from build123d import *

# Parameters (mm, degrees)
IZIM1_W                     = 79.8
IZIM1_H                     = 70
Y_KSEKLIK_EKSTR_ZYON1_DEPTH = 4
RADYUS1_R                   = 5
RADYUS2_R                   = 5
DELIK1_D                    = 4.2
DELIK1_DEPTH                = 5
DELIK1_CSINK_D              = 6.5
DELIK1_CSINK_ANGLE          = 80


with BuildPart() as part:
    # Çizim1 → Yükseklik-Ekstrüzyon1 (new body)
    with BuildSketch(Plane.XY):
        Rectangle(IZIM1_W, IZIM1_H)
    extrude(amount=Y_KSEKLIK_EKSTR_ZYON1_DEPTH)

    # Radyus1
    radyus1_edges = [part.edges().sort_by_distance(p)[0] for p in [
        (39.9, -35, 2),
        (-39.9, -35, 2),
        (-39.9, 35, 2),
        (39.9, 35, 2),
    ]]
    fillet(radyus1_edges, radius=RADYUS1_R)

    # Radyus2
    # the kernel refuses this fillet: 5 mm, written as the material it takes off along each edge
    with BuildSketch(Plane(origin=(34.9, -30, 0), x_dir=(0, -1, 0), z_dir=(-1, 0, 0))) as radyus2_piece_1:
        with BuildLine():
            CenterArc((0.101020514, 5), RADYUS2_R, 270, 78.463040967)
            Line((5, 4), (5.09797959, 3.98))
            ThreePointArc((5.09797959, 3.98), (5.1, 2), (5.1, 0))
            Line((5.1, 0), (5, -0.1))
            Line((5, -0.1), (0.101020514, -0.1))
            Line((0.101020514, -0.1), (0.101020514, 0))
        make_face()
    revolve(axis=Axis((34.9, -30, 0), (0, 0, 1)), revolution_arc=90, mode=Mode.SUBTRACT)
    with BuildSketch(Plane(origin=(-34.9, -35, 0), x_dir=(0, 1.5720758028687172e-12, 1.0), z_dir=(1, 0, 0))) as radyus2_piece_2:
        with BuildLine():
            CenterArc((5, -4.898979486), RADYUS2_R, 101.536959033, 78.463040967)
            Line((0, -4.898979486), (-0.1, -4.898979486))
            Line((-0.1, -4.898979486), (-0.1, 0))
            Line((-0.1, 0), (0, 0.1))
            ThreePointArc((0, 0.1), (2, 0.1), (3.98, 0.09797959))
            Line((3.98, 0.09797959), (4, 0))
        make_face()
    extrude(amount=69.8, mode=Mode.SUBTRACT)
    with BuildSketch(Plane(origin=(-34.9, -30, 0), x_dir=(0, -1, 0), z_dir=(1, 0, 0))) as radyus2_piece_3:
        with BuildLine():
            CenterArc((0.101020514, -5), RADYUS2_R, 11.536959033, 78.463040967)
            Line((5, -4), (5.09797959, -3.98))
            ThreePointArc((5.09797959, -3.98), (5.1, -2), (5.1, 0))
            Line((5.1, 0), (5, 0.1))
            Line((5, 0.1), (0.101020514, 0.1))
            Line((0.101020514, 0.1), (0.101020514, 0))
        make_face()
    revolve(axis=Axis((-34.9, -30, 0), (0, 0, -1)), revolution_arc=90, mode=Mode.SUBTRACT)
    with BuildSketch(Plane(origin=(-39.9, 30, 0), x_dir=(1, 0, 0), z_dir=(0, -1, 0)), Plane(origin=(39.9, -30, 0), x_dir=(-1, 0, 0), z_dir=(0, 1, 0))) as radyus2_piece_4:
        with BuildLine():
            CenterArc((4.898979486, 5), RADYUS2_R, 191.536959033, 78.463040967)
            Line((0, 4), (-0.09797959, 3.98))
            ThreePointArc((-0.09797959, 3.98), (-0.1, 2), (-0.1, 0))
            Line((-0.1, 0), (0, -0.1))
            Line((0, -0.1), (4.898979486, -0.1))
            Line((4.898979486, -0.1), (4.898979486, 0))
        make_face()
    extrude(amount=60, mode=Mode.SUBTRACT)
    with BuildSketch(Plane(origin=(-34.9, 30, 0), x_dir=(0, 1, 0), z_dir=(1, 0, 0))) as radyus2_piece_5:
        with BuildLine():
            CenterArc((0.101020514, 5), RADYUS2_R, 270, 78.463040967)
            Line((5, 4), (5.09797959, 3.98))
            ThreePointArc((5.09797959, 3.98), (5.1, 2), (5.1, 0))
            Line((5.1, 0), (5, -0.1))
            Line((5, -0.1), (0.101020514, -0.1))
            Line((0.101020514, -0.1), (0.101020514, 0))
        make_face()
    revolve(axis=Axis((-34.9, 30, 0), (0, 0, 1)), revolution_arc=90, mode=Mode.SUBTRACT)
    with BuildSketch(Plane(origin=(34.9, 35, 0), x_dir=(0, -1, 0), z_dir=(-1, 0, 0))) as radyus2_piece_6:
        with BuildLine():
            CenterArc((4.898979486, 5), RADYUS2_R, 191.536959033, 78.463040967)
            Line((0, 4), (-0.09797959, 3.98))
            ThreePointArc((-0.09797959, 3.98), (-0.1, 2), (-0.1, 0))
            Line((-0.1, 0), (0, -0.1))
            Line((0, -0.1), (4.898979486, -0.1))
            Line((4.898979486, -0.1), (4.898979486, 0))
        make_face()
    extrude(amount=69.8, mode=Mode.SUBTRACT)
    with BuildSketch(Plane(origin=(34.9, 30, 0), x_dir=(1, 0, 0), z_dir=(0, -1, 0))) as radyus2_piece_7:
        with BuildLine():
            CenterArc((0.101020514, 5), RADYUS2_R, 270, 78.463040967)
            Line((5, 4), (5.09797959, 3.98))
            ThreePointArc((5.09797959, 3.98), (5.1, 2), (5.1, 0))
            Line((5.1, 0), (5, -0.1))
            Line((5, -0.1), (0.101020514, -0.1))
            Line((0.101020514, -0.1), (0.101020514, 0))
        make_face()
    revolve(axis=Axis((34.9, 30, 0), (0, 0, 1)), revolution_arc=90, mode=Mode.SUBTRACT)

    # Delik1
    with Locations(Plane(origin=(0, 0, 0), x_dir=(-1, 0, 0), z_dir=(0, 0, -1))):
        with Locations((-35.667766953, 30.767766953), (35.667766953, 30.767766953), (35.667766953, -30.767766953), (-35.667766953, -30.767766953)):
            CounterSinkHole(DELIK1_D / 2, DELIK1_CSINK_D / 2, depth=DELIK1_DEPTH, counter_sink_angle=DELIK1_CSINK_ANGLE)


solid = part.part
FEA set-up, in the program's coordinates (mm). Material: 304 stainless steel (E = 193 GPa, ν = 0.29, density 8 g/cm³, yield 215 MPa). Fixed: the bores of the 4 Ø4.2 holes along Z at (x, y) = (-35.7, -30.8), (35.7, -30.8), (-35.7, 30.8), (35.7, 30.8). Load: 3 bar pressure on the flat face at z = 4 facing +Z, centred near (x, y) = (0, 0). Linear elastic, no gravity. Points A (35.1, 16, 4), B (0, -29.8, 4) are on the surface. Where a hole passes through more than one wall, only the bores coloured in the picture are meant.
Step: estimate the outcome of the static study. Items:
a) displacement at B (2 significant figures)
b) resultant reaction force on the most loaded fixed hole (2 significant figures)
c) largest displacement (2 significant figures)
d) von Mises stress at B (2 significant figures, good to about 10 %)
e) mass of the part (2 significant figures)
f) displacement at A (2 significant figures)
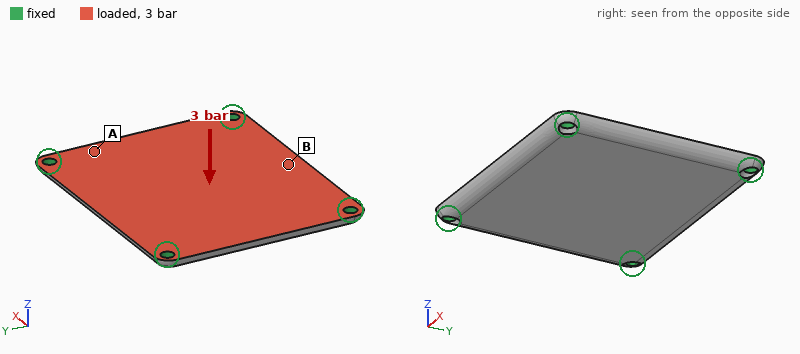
42 µm
520 N
56 µm
38 MPa
170 g
15 µm
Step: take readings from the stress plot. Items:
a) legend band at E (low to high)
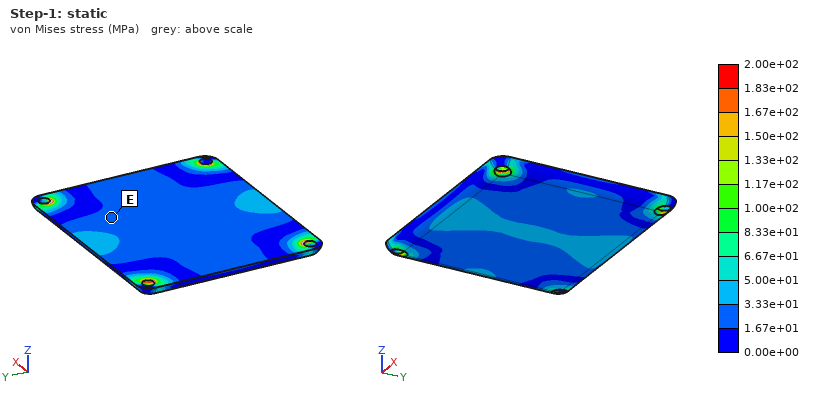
1.67e+01 to 3.33e+01 MPa
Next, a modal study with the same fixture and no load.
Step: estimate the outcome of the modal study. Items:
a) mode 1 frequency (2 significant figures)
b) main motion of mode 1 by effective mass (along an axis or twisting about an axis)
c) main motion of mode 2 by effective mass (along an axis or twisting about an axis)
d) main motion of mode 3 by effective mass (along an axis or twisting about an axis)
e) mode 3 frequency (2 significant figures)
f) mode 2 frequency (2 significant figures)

2500 Hz
along Z
twisting about X
twisting about Y
4900 Hz
4300 Hz
